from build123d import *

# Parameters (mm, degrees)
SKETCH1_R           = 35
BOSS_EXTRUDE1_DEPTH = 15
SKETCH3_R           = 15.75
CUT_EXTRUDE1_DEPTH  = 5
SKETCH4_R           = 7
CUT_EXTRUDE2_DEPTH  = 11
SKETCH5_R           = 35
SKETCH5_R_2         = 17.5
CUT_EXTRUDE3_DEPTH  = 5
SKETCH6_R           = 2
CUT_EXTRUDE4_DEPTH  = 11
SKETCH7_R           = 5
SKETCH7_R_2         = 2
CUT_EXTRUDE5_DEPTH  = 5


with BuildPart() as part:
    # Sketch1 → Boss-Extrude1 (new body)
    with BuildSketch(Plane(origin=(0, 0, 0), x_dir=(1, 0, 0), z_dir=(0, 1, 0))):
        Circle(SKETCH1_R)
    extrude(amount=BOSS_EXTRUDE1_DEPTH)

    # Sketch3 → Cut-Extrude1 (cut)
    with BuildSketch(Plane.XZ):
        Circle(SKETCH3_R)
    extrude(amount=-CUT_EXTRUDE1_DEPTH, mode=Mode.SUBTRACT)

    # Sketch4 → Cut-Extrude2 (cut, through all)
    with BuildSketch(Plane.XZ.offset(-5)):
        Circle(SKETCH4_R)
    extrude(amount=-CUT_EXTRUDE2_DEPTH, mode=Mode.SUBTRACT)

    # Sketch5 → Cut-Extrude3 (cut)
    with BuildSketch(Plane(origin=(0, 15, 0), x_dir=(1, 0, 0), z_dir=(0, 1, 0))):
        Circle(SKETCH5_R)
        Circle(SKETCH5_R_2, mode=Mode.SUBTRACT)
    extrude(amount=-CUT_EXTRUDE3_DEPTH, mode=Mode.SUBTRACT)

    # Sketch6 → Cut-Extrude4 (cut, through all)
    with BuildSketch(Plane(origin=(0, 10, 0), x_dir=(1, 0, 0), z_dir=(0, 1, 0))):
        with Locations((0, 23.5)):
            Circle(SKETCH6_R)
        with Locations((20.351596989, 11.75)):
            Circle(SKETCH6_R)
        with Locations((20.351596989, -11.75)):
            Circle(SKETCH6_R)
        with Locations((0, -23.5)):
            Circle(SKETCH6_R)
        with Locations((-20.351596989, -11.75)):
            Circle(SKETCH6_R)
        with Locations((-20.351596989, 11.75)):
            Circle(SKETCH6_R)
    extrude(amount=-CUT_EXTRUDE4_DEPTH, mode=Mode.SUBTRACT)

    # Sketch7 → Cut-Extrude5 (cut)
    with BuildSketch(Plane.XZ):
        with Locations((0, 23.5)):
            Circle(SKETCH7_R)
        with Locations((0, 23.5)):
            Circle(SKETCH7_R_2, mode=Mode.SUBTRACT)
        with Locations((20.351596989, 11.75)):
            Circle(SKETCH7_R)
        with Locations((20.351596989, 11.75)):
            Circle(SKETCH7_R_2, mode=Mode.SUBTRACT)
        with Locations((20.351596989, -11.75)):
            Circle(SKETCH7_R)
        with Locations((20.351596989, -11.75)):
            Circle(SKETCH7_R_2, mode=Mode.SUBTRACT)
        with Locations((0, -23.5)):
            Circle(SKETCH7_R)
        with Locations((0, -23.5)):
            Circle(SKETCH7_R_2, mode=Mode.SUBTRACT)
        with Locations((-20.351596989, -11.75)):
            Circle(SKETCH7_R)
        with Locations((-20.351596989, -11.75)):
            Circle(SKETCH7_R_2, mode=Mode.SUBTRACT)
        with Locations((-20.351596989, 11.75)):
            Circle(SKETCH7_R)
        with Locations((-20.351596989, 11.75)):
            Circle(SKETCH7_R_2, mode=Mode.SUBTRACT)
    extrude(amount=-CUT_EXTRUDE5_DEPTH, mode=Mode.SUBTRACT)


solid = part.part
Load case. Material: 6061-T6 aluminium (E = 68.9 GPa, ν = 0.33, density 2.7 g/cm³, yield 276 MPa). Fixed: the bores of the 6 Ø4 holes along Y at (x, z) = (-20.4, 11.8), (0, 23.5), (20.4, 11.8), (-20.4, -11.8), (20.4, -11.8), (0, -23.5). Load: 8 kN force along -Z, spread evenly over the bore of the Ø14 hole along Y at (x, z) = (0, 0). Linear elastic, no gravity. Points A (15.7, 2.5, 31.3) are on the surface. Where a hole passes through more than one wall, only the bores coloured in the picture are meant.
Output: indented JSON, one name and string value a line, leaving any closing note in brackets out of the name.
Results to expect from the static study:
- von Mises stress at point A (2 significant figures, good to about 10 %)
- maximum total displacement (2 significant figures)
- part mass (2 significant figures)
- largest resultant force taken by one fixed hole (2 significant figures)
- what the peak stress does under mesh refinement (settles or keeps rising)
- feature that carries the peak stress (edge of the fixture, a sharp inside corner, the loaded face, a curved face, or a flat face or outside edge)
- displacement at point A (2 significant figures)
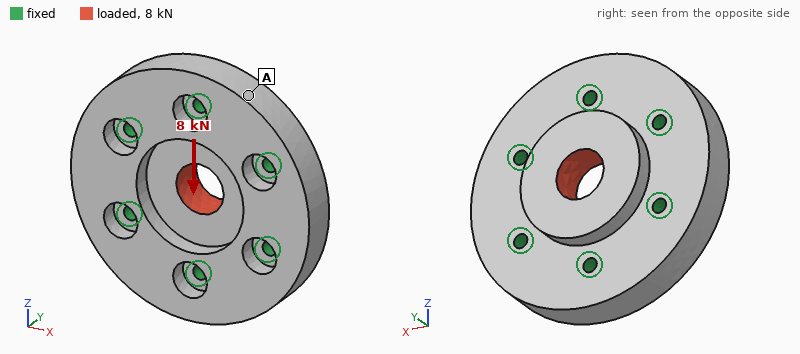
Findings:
{
  "von Mises stress at point A": "4.7 MPa",
  "maximum total displacement": "7.6 µm",
  "part mass": "95 g",
  "largest resultant force taken by one fixed hole": "1.9 kN",
  "what the peak stress does under mesh refinement": "keeps rising",
  "feature that carries the peak stress": "edge of the fixture",
  "displacement at point A": "1.7 µm"
}
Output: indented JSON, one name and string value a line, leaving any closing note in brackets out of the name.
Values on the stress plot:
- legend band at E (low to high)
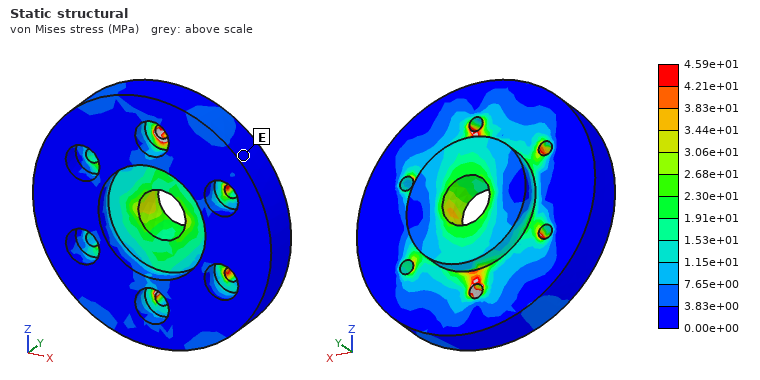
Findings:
{
  "legend band at E": "0.00e+00 to 3.83e+00 MPa"
}
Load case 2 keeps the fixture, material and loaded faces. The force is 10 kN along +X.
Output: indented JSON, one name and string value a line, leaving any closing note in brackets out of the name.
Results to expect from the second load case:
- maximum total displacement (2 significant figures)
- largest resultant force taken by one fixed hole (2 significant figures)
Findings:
{
  "maximum total displacement": "9.5 µm",
  "largest resultant force taken by one fixed hole": "2.1 kN"
}
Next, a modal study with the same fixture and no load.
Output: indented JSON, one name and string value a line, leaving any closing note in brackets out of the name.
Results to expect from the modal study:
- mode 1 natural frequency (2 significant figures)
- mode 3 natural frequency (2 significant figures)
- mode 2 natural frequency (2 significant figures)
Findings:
{
  "mode 1 natural frequency": "19 kHz",
  "mode 3 natural frequency": "20 kHz",
  "mode 2 natural frequency": "20 kHz"
}
